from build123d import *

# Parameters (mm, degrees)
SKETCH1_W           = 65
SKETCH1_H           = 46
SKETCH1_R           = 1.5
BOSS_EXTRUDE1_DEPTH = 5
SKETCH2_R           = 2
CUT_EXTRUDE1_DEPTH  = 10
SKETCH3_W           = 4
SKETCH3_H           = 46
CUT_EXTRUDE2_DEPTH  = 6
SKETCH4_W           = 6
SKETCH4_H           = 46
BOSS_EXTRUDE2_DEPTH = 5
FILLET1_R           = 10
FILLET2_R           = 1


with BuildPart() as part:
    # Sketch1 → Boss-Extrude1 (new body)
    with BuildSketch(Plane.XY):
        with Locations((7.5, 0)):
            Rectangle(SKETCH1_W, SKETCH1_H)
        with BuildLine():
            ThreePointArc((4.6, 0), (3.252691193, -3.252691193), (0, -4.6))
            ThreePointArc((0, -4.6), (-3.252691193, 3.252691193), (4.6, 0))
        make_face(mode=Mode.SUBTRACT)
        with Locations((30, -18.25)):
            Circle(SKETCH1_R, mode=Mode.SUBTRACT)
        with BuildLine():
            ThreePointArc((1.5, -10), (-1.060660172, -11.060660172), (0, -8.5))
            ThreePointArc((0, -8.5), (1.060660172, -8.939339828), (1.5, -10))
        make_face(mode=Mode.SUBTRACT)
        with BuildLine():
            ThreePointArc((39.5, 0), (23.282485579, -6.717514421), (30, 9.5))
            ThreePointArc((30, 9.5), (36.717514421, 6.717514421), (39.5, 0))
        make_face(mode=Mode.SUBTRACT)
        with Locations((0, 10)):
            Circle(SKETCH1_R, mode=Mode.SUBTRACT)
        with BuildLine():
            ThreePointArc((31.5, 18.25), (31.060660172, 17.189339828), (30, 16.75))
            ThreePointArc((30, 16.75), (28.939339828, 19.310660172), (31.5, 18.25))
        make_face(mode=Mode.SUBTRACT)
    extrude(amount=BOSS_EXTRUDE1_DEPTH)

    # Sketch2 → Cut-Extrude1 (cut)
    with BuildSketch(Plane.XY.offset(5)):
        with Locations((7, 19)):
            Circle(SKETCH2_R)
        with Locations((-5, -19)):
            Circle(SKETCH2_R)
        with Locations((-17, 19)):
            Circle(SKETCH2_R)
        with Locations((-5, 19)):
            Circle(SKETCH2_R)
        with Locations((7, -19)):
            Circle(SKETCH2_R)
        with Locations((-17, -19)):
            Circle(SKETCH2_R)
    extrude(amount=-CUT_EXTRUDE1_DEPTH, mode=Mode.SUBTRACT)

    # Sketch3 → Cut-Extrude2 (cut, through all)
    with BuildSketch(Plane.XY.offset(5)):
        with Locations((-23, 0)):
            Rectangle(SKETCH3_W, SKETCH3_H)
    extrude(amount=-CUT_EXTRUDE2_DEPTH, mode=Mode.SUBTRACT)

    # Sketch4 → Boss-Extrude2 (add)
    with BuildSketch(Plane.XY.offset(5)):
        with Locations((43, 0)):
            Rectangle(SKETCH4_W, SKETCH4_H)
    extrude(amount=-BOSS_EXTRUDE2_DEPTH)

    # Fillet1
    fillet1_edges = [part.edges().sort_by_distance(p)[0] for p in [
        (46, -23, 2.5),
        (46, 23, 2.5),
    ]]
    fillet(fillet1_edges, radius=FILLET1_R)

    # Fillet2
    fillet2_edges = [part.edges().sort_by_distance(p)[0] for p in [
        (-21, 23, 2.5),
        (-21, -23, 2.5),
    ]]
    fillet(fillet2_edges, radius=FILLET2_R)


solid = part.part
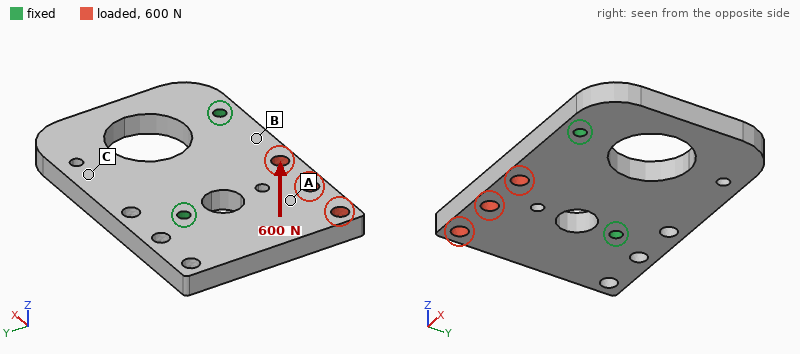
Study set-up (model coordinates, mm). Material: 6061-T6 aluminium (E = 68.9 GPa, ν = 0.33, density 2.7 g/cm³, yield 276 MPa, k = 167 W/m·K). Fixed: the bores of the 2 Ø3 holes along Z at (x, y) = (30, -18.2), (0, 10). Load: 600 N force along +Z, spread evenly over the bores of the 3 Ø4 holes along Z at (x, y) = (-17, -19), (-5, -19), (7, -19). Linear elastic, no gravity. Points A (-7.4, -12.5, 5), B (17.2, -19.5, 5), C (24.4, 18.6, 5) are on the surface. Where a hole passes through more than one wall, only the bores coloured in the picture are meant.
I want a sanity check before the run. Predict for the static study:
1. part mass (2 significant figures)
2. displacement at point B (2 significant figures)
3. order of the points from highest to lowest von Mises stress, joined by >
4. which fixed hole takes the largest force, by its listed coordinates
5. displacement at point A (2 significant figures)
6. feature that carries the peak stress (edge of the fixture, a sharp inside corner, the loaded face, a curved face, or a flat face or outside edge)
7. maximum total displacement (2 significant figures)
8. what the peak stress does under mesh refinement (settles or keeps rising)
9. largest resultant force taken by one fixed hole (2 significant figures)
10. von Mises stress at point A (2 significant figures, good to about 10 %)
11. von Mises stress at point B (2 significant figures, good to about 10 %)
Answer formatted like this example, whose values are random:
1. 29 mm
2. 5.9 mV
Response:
1. 35 g
2. 0.046 mm
3. B > A > C
4. (0, 10)
5. 0.15 mm
6. edge of the fixture
7. 0.31 mm
8. keeps rising
9. 350 N
10. 32 MPa
11. 58 MPa
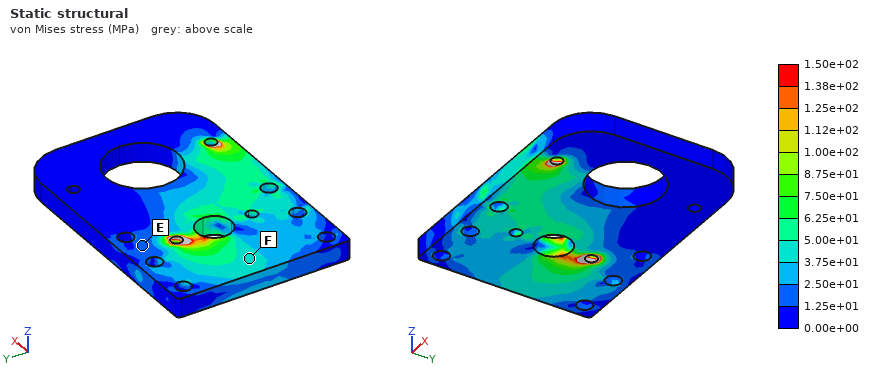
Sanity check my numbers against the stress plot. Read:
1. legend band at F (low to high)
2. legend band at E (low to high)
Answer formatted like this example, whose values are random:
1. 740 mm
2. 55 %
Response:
1. 3.75e+01 to 5.00e+01 MPa
2. 1.25e+01 to 2.50e+01 MPa
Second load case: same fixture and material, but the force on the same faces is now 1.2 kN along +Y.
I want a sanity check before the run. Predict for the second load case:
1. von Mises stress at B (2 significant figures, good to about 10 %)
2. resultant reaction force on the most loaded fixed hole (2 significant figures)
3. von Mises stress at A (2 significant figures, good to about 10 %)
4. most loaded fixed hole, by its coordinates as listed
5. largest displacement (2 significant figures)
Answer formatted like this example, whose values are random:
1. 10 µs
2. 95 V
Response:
1. 5.1 MPa
2. 1.1 kN
3. 8.6 MPa
4. (0, 10)
5. 11 µm
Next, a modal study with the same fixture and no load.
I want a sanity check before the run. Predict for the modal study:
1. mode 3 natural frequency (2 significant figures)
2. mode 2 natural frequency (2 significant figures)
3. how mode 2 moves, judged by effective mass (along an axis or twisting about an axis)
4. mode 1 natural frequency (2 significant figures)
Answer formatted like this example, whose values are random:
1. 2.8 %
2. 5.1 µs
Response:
1. 7800 Hz
2. 4000 Hz
3. along Z
4. 3100 Hz
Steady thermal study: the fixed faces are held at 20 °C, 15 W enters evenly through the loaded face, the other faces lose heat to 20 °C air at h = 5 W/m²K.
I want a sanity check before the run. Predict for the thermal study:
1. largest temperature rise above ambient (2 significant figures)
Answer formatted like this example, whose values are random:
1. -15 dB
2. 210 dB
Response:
1. 19 K
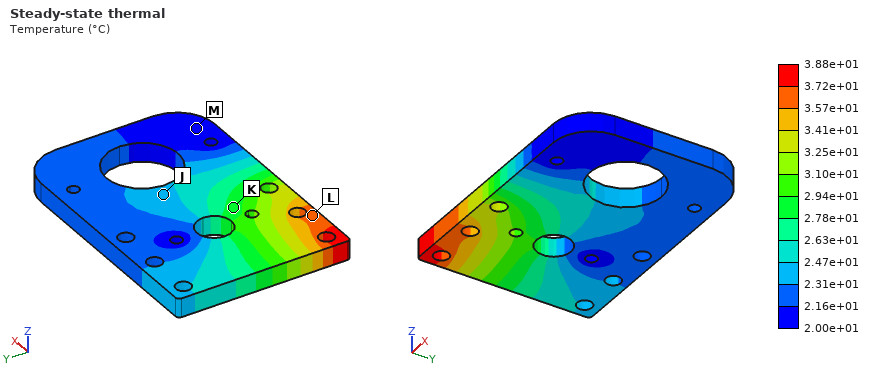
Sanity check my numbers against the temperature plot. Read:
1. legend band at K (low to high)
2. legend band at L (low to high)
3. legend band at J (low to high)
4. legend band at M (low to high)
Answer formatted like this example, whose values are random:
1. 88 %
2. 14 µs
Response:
1. 2.78e+01 to 2.94e+01 °C
2. 3.57e+01 to 3.72e+01 °C
3. 2.31e+01 to 2.47e+01 °C
4. 2.00e+01 to 2.16e+01 °C
